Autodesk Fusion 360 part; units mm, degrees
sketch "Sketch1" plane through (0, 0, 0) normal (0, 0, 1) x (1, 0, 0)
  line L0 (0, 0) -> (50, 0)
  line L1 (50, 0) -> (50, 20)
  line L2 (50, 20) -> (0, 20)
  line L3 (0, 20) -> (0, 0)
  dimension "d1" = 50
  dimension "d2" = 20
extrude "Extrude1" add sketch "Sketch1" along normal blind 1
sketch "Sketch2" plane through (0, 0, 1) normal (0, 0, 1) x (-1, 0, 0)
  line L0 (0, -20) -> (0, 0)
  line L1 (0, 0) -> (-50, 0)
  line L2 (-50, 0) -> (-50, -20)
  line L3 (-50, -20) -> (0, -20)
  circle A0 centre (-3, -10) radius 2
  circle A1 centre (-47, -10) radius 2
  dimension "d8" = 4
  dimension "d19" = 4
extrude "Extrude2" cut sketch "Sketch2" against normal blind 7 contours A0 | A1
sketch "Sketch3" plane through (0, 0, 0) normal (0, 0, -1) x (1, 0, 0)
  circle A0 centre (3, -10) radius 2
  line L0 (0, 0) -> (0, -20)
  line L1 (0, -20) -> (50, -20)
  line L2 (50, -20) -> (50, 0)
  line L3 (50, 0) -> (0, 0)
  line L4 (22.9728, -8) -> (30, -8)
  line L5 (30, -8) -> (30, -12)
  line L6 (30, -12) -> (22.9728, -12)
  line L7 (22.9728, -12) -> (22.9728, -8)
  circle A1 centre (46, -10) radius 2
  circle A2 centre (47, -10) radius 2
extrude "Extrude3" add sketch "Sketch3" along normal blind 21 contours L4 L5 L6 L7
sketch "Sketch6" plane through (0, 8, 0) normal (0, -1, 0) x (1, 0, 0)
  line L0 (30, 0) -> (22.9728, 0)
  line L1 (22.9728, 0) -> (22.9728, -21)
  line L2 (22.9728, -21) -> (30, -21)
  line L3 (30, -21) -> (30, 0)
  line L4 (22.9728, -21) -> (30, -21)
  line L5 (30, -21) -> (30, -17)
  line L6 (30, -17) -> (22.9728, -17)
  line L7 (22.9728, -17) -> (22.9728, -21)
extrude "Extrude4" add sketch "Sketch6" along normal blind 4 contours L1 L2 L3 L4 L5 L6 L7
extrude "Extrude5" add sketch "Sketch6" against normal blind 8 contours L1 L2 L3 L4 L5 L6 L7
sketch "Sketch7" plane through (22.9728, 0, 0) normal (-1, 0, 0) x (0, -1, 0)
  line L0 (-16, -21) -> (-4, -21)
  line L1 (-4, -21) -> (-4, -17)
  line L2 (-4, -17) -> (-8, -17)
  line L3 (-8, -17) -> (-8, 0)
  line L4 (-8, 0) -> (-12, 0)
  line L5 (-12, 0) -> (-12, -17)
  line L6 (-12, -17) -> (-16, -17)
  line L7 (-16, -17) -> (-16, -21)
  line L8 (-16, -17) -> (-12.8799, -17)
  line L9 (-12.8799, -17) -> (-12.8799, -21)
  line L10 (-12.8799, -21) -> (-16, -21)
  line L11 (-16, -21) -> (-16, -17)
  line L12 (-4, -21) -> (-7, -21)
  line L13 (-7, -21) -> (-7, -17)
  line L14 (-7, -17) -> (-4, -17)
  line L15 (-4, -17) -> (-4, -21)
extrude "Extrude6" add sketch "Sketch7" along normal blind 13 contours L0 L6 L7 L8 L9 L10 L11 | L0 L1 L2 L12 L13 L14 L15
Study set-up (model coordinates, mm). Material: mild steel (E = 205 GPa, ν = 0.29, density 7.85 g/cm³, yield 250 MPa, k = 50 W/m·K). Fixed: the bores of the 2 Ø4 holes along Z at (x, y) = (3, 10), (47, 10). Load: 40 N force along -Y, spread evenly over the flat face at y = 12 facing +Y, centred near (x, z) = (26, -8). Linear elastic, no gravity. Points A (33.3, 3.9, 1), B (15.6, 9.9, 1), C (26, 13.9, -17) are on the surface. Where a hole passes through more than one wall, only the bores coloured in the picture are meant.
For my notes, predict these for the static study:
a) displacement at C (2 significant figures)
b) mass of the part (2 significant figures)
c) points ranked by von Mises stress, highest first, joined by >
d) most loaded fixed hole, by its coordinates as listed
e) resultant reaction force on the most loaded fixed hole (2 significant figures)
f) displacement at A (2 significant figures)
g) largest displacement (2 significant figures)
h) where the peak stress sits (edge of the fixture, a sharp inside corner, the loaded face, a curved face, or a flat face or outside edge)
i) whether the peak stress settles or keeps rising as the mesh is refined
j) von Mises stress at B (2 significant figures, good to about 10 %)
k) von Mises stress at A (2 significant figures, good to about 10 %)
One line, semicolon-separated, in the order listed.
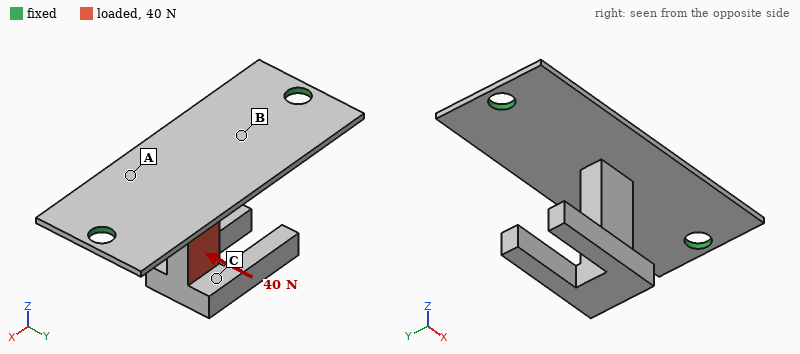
0.12 mm; 17 g; B > A > C; (47, 10); 22 N; 0.028 mm; 0.14 mm; edge of the fixture; keeps rising; 42 MPa; 27 MPa
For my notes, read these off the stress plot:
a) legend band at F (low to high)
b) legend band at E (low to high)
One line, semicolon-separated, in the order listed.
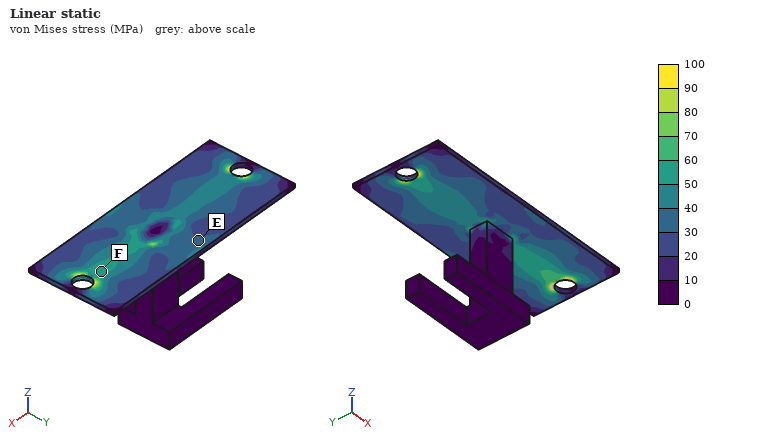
50 to 60 MPa; 30 to 40 MPa
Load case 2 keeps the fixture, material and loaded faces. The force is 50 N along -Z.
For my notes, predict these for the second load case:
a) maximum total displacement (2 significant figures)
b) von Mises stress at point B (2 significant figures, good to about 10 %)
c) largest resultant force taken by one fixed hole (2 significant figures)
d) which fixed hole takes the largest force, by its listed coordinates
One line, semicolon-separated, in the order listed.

75 µm; 17 MPa; 28 N; (47, 10)
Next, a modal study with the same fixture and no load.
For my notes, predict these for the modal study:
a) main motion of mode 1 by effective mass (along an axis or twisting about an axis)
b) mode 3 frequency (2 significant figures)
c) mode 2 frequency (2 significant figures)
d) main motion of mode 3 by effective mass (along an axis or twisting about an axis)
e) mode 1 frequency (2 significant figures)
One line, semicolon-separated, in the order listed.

along Y; 1700 Hz; 1200 Hz; along Z; 740 Hz
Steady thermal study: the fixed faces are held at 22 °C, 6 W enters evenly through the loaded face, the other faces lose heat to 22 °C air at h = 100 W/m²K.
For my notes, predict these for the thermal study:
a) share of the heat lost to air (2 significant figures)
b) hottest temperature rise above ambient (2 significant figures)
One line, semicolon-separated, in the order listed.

77 %; 39 K
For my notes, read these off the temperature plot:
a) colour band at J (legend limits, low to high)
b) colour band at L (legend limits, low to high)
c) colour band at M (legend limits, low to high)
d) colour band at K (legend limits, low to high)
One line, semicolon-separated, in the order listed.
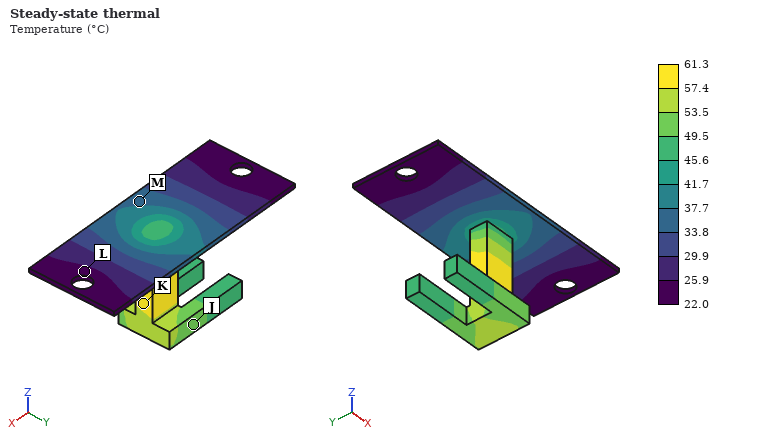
49.5 to 53.5 °C; 22.0 to 25.9 °C; 33.8 to 37.7 °C; 57.4 to 61.3 °C
